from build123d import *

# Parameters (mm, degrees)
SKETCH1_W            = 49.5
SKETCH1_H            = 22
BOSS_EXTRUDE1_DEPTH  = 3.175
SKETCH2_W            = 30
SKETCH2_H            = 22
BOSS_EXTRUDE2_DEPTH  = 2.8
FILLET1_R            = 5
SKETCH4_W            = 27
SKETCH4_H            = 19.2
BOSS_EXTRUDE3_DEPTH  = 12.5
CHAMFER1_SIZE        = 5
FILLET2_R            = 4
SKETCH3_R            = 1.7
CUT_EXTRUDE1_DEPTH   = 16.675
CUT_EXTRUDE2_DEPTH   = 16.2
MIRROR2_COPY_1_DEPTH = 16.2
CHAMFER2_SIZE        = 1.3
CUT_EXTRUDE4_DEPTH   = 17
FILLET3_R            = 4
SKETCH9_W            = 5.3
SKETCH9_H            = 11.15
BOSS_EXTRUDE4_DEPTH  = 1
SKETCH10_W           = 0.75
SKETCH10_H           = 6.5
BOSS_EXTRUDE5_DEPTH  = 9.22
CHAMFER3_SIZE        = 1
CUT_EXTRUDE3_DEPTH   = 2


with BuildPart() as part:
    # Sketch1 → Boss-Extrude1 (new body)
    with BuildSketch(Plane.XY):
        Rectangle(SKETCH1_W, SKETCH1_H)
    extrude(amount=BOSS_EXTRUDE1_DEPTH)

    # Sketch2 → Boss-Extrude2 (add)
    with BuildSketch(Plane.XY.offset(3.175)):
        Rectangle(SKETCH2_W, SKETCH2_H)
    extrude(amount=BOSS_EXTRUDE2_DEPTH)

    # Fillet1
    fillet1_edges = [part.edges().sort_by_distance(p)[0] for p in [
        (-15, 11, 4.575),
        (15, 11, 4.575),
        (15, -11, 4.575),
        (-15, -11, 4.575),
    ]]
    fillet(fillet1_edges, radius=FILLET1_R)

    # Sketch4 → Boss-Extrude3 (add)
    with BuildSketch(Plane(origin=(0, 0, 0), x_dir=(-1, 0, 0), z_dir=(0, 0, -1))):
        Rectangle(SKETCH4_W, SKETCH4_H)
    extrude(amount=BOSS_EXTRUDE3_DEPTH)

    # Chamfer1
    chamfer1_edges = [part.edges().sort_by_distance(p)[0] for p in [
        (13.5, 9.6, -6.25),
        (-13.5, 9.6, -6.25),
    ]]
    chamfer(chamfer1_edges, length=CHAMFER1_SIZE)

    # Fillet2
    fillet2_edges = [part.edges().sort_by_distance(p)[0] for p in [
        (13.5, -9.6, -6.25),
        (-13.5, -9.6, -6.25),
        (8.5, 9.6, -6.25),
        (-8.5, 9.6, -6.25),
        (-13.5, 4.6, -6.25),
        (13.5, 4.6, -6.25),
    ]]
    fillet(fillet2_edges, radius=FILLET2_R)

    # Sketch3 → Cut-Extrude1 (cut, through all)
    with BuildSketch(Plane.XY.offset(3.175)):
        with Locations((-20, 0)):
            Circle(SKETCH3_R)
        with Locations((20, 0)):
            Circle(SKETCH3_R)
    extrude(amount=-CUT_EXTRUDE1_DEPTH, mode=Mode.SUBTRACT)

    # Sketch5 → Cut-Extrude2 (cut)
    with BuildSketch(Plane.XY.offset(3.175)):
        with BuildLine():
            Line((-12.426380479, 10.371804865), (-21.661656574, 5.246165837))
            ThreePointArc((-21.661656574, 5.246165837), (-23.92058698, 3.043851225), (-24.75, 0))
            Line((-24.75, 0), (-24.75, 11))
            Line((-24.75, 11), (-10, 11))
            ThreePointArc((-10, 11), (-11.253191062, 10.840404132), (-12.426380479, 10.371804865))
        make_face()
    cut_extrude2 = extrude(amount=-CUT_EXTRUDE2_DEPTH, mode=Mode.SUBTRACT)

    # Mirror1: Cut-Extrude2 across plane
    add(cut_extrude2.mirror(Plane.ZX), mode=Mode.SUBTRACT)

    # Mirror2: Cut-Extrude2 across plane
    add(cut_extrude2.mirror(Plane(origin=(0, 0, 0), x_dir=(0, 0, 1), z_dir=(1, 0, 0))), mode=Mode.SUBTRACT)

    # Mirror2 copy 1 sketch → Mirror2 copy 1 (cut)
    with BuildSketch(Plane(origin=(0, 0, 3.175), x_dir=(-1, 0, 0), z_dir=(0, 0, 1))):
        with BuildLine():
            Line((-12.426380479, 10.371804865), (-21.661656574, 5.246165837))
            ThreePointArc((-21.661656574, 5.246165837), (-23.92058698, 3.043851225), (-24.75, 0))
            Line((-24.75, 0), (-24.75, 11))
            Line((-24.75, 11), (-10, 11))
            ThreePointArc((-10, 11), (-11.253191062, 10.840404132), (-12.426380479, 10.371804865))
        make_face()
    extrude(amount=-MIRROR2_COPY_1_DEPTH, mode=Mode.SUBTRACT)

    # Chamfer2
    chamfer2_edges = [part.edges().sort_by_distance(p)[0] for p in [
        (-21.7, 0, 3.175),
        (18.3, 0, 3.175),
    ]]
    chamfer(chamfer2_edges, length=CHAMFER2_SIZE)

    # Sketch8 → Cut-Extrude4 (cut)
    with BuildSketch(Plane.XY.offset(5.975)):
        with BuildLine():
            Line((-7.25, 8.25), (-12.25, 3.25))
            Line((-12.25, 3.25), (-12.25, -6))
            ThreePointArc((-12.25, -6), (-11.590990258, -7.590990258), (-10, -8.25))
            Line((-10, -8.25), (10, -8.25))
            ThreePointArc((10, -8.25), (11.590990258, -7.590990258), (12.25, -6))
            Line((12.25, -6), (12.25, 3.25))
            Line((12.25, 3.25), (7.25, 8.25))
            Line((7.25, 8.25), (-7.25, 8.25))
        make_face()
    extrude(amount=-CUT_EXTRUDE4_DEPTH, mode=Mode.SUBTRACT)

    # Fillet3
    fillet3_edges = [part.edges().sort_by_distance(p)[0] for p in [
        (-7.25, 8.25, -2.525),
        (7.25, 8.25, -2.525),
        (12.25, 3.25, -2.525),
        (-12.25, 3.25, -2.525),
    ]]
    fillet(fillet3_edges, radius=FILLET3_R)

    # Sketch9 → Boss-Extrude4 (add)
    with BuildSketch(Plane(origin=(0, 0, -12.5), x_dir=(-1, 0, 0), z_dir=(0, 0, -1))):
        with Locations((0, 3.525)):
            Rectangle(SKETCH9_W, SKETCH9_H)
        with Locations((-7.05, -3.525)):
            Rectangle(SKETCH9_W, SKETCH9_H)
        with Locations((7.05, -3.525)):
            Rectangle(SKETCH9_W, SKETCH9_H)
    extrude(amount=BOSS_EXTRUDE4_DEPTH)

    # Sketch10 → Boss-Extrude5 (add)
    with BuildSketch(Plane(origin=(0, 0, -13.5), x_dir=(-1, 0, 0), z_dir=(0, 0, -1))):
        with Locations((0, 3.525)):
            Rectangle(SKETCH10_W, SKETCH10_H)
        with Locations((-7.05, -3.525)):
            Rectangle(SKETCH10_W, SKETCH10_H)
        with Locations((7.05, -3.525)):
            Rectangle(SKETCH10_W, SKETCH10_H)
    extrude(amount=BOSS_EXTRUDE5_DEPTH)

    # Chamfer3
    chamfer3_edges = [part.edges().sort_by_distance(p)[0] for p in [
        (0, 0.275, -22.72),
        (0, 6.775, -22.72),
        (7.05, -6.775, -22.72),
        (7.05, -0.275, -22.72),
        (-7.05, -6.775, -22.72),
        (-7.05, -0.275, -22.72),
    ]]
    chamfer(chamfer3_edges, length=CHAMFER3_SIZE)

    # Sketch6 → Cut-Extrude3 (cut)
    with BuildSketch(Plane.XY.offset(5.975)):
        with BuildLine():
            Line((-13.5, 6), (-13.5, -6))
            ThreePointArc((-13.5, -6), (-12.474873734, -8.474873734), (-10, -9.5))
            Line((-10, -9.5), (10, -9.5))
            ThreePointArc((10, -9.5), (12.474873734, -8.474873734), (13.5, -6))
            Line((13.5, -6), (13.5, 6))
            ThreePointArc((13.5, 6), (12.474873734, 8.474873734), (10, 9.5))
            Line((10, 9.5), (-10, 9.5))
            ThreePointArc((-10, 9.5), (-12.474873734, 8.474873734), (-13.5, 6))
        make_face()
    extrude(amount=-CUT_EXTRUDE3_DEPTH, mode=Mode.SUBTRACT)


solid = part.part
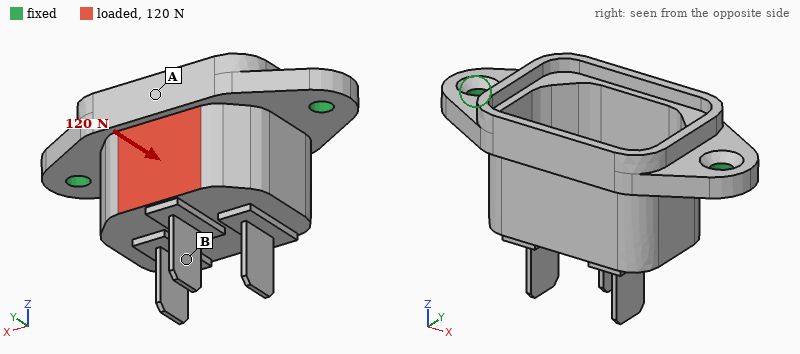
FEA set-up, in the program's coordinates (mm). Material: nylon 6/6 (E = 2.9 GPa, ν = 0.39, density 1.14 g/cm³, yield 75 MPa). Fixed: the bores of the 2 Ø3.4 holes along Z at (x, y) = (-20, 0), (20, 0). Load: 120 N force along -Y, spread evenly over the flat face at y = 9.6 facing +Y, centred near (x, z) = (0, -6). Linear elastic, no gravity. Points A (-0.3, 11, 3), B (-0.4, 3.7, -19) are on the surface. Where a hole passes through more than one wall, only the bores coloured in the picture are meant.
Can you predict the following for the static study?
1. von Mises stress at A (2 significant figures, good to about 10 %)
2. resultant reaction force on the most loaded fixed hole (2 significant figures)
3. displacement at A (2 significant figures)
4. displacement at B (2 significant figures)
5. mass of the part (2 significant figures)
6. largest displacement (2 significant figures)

7.3 MPa
69 N
0.28 mm
0.52 mm
4.8 g
0.62 mm
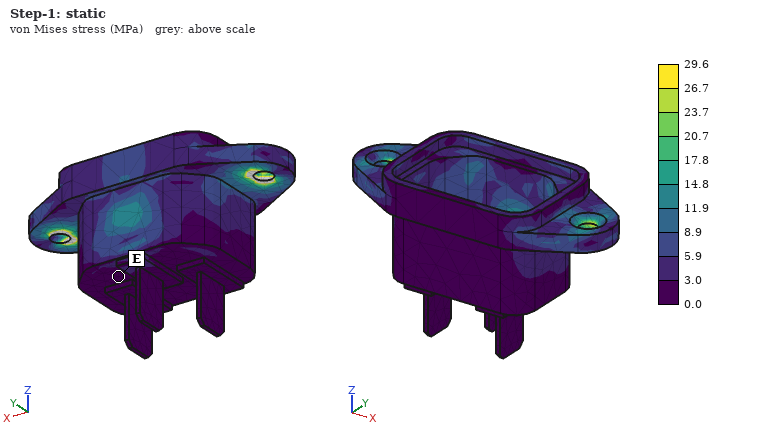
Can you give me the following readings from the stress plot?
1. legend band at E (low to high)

0.0 to 3.0 MPa
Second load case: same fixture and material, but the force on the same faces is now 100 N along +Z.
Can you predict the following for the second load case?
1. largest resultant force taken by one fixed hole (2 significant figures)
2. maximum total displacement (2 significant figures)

52 N
0.66 mm
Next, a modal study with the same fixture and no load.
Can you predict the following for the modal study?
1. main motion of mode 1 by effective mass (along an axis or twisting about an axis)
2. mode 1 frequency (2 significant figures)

along Y
1300 Hz
